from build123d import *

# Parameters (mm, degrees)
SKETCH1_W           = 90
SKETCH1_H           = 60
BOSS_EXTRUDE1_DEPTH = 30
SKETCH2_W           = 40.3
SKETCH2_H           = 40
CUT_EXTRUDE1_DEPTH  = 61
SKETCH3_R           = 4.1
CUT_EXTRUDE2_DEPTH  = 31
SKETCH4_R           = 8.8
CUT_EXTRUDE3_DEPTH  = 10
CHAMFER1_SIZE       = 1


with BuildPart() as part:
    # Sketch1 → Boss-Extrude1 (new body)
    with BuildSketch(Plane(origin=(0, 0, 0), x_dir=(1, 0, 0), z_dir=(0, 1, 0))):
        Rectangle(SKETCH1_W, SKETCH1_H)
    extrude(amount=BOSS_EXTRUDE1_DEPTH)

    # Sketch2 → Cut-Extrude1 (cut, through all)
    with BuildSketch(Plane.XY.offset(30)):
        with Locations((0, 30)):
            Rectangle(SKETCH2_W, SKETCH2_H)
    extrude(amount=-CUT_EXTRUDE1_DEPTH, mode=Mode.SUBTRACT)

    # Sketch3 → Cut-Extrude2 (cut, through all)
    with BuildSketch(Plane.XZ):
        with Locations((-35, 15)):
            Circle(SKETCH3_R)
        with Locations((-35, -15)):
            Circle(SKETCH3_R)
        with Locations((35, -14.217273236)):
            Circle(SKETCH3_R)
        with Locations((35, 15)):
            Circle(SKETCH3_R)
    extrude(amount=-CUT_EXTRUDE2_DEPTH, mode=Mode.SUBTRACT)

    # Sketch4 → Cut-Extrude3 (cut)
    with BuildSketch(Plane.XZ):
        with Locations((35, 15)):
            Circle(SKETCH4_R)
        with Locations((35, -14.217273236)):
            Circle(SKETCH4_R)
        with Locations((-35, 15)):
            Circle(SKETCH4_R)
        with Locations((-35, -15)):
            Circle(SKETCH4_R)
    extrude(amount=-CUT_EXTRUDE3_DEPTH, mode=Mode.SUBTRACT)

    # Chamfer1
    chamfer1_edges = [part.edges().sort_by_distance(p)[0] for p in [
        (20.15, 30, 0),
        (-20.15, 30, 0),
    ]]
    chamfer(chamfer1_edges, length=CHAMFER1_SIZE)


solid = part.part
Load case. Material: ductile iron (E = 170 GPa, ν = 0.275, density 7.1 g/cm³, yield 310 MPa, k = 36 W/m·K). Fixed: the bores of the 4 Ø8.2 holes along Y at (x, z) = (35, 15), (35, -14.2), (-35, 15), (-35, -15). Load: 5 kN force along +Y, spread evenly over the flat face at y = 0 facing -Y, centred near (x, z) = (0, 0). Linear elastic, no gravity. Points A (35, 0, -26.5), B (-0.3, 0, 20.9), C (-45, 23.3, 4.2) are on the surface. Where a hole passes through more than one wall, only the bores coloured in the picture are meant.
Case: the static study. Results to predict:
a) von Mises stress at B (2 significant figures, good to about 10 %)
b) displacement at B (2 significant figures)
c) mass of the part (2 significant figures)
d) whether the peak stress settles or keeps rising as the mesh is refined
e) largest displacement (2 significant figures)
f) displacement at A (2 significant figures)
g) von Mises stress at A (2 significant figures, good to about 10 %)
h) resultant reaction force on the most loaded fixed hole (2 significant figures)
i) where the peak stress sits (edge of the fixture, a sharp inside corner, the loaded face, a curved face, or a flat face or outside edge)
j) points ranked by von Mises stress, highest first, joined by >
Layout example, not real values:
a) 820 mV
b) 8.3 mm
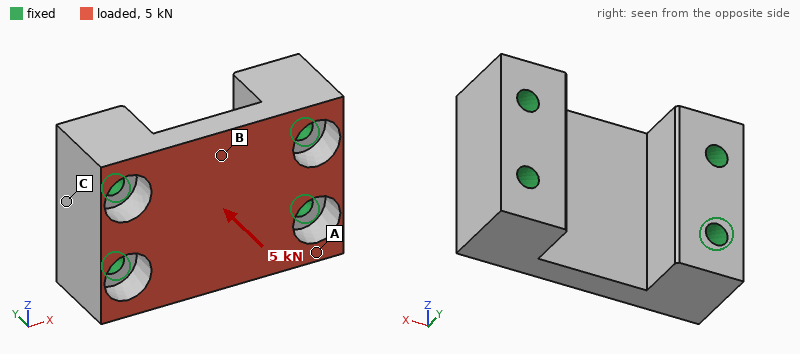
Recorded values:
a) 8.5 MPa
b) 2.4 µm
c) 710 g
d) keeps rising
e) 2.7 µm
f) 0.44 µm
g) 2.4 MPa
h) 1.4 kN
i) edge of the fixture
j) B > A > C
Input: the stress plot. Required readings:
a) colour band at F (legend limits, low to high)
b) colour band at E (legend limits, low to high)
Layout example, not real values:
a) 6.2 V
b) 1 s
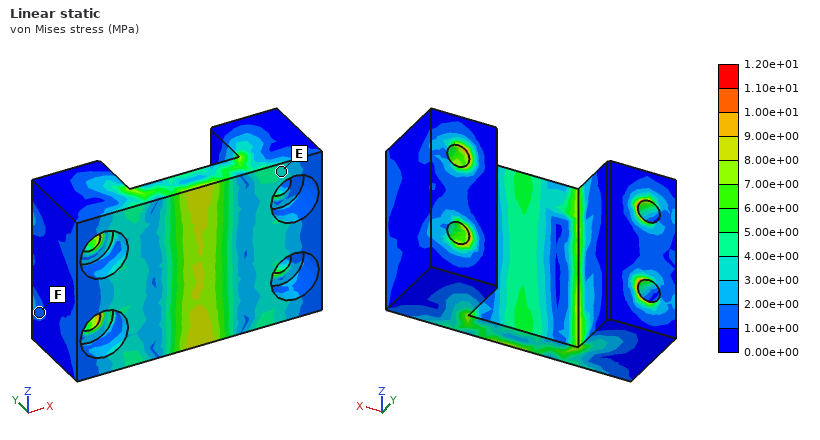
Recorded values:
a) 1.00e+00 to 2.00e+00 MPa
b) 3.00e+00 to 4.00e+00 MPa
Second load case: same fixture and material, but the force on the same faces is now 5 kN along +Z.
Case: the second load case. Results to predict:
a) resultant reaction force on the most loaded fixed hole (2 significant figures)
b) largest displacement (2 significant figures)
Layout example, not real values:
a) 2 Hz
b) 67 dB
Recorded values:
a) 1.7 kN
b) 2.8 µm
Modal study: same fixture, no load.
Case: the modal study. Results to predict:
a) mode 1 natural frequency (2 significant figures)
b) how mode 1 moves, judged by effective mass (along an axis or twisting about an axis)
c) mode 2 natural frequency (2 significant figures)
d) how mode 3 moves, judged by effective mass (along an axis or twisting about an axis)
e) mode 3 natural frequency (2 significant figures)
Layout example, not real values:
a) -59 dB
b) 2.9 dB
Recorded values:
a) 14 kHz
b) along Y
c) 15 kHz
d) along X
e) 18 kHz
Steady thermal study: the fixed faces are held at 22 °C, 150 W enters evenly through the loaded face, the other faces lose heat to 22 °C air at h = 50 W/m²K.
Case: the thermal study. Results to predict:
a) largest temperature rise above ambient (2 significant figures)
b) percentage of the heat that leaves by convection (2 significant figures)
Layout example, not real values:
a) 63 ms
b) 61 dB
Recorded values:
a) 57 K
b) 10 %
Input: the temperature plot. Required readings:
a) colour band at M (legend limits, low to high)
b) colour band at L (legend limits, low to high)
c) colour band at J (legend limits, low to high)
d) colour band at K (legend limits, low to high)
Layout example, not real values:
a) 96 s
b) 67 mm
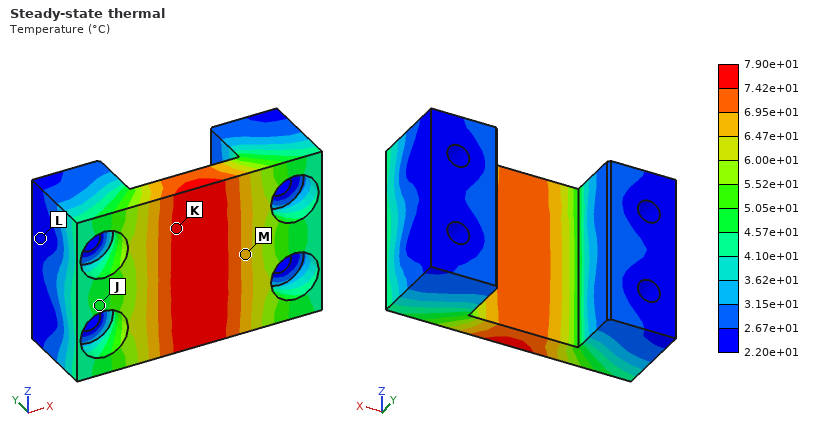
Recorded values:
a) 6.47e+01 to 6.95e+01 °C
b) 2.20e+01 to 2.67e+01 °C
c) 4.57e+01 to 5.05e+01 °C
d) 7.42e+01 to 7.90e+01 °C
